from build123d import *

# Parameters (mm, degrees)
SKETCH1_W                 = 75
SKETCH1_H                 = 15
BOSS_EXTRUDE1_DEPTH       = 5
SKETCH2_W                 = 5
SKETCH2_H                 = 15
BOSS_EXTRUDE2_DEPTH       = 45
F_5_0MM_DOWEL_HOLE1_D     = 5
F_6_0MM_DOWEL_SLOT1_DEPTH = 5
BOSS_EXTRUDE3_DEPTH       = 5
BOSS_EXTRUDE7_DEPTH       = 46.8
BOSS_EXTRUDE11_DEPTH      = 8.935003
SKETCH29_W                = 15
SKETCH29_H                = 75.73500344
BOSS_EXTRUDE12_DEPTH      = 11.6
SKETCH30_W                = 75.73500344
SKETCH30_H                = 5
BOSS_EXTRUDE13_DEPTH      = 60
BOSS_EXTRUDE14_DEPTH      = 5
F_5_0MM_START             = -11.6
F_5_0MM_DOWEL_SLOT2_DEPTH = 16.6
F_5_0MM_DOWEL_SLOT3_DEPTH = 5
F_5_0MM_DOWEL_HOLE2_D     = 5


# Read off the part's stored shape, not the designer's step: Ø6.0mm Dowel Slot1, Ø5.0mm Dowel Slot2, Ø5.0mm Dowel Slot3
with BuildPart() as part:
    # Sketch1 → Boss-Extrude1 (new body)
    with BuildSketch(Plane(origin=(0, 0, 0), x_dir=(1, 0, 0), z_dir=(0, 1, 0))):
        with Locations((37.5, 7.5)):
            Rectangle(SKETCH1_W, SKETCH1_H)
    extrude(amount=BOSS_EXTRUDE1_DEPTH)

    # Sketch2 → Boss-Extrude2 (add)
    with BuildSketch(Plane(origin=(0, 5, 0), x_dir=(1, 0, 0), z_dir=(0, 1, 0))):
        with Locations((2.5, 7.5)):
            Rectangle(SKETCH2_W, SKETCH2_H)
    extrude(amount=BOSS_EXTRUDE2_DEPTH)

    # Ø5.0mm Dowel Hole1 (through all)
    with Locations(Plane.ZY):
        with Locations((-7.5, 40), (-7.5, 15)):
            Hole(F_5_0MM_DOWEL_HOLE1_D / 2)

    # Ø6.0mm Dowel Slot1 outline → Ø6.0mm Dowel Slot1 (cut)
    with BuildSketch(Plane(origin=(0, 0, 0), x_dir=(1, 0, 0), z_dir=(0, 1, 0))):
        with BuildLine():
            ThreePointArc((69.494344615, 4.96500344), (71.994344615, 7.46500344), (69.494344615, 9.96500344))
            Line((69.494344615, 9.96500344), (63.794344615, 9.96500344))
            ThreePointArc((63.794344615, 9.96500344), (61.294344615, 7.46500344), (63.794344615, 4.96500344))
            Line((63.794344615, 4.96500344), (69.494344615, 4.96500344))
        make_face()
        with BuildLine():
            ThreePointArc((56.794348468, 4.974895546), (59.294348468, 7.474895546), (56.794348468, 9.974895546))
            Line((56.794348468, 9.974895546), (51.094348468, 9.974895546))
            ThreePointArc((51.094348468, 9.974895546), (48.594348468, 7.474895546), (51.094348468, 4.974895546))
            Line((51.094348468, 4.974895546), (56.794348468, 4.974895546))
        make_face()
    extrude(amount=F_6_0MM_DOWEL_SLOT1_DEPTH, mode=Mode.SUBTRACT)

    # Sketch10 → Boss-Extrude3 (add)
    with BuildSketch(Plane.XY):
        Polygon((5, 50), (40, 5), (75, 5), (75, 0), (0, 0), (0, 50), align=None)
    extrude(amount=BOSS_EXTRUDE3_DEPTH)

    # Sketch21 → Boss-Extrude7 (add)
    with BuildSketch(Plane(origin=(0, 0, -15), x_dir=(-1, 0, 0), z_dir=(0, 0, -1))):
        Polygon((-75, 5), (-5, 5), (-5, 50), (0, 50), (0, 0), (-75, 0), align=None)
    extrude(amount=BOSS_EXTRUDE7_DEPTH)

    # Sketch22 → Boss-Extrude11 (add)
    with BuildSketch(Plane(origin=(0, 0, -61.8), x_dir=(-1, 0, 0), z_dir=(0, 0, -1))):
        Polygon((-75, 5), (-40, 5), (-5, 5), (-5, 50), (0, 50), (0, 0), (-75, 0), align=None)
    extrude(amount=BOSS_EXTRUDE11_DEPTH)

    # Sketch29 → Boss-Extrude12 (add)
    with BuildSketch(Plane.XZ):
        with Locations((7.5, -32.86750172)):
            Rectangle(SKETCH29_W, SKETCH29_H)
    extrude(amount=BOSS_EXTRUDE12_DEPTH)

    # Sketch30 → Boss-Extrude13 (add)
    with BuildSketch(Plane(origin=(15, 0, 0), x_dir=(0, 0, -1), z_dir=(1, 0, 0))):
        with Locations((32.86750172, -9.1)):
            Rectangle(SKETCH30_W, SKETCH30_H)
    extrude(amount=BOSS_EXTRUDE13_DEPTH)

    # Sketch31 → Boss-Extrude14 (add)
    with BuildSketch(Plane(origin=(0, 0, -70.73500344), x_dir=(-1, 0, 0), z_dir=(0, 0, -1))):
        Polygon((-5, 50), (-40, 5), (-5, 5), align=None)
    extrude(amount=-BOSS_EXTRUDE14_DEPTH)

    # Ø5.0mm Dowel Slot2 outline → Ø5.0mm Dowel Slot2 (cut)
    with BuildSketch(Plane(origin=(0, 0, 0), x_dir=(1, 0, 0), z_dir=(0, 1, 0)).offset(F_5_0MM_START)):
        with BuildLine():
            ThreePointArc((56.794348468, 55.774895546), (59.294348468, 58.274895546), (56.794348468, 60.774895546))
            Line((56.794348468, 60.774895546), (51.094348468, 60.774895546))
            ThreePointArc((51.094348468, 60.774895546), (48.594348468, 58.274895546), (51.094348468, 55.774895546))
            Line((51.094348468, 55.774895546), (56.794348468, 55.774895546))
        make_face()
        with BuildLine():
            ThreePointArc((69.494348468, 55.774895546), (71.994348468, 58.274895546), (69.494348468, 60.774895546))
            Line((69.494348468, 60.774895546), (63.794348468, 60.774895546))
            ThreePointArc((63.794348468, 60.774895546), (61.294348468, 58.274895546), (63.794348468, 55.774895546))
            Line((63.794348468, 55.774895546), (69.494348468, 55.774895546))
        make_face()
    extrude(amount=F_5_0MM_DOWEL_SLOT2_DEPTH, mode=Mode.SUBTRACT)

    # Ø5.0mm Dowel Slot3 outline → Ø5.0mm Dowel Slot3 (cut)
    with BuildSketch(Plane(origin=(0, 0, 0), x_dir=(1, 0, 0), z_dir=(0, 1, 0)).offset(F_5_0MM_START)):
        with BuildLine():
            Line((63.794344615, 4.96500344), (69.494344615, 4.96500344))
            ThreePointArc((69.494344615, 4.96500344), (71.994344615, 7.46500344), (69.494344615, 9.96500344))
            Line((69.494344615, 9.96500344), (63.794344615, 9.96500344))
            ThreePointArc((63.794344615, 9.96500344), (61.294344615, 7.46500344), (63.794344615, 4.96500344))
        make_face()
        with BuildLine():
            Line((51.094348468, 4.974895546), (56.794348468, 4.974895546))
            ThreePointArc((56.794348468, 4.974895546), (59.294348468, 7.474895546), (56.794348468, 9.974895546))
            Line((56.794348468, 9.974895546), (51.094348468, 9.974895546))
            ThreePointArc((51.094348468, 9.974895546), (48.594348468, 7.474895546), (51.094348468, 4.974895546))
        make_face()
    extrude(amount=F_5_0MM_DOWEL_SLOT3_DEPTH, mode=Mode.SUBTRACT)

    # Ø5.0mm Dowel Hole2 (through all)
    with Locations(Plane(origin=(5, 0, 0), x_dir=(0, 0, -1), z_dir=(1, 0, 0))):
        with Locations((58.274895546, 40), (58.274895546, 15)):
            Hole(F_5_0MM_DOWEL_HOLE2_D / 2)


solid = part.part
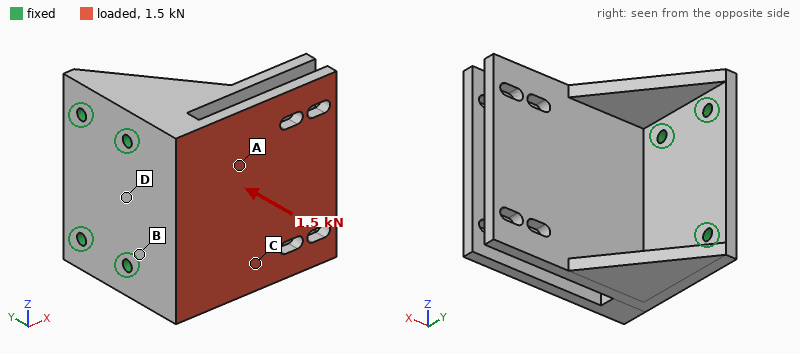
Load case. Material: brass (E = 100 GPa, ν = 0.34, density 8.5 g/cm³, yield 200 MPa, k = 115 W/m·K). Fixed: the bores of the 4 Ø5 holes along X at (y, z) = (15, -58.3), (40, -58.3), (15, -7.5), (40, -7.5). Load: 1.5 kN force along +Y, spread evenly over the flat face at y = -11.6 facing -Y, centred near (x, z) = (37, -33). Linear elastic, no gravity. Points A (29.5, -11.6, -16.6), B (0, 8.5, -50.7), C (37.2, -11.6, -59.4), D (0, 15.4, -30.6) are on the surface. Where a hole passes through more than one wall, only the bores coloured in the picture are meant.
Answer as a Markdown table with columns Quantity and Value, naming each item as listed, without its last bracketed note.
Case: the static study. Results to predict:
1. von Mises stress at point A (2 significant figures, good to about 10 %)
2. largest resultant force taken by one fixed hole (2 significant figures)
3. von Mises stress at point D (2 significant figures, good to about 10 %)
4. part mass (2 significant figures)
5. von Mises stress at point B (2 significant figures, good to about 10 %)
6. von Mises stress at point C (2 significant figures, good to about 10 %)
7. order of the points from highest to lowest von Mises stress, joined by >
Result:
| Quantity | Value |
|---|---|
| von Mises stress at point A | 56 MPa |
| largest resultant force taken by one fixed hole | 1.0 kN |
| von Mises stress at point D | 17 MPa |
| part mass | 740 g |
| von Mises stress at point B | 29 MPa |
| von Mises stress at point C | 42 MPa |
| order of the points from highest to lowest von Mises stress, joined by > | A > C > B > D |
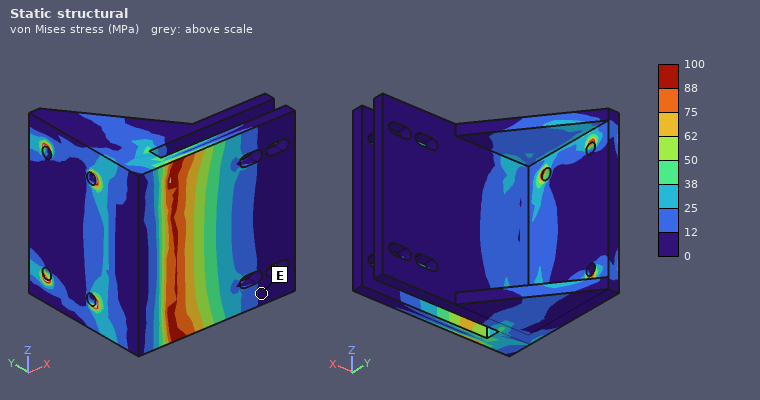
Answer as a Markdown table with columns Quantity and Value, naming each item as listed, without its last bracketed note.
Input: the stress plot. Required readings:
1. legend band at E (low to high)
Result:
| Quantity | Value |
|---|---|
| legend band at E | 0 to 12 MPa |
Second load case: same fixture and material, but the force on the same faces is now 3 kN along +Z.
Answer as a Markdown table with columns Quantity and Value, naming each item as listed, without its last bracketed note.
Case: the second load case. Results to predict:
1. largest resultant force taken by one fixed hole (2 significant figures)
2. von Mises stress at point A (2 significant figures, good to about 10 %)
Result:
| Quantity | Value |
|---|---|
| largest resultant force taken by one fixed hole | 2.9 kN |
| von Mises stress at point A | 12 MPa |
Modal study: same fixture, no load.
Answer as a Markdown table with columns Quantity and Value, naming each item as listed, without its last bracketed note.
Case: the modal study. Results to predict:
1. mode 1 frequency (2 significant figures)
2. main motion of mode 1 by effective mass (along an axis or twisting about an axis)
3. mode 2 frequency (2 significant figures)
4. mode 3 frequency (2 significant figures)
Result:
| Quantity | Value |
|---|---|
| mode 1 frequency | 650 Hz |
| main motion of mode 1 by effective mass | along Y |
| mode 2 frequency | 1000 Hz |
| mode 3 frequency | 1400 Hz |
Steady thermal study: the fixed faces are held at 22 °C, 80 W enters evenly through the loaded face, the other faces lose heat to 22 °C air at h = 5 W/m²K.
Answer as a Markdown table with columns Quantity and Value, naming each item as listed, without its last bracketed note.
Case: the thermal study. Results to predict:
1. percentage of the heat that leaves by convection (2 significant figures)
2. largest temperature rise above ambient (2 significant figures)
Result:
| Quantity | Value |
|---|---|
| percentage of the heat that leaves by convection | 5.0 % |
| largest temperature rise above ambient | 79 K |
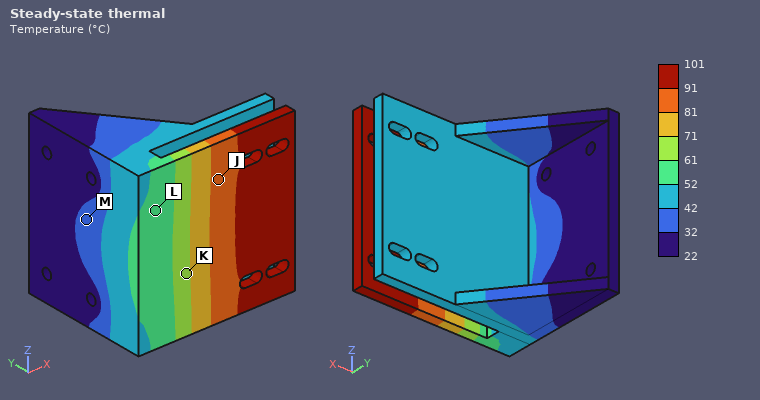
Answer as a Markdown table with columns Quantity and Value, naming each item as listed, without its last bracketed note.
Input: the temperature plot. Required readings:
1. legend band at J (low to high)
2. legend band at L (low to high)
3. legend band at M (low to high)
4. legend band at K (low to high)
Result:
| Quantity | Value |
|---|---|
| legend band at J | 81 to 91 °C |
| legend band at L | 52 to 61 °C |
| legend band at M | 32 to 42 °C |
| legend band at K | 61 to 71 °C |
